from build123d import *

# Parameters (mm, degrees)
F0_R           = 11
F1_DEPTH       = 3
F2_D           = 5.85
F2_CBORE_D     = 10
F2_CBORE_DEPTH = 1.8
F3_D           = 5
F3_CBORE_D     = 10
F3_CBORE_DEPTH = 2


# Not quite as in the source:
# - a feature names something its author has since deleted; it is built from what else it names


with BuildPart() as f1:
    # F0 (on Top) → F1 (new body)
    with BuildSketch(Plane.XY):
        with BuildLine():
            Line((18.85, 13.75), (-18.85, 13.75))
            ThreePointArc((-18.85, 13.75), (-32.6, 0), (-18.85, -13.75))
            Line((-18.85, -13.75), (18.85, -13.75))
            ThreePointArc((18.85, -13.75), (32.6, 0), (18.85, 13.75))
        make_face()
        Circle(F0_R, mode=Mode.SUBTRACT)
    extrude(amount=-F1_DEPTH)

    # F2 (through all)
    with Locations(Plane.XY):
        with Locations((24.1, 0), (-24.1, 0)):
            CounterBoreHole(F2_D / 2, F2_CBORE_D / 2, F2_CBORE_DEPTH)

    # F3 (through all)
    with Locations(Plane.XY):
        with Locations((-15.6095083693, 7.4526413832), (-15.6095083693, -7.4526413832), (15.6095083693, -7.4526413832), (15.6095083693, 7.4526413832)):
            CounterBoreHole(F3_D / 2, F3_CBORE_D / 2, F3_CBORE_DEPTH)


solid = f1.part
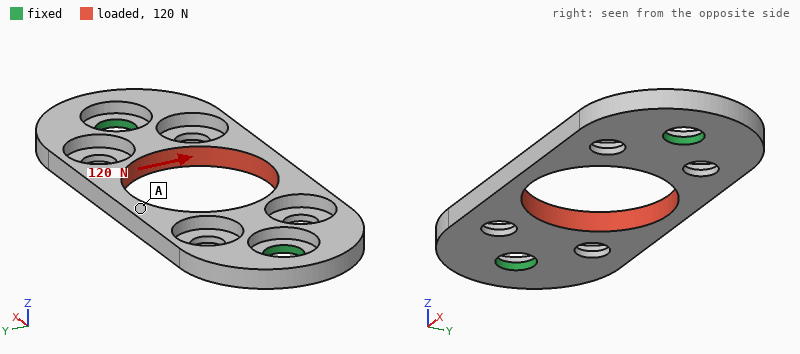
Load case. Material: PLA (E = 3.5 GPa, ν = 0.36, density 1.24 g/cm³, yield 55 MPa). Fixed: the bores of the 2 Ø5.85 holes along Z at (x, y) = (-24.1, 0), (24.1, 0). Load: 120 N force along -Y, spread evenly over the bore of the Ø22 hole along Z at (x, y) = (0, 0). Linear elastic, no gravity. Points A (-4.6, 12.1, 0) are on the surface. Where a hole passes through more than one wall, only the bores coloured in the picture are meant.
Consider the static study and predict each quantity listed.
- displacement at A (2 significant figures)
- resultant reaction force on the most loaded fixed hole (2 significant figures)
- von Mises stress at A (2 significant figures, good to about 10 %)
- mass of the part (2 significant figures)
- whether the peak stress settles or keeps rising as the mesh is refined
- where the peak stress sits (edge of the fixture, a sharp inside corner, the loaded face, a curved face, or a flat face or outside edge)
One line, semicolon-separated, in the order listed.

0.097 mm; 60 N; 1.7 MPa; 3.3 g; keeps rising; edge of the fixture
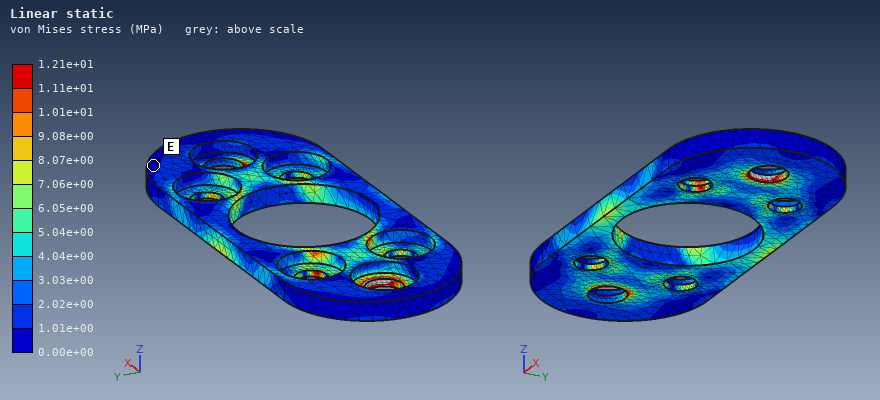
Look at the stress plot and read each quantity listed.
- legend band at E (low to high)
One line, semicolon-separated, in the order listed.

0.00e+00 to 1.01e+00 MPa
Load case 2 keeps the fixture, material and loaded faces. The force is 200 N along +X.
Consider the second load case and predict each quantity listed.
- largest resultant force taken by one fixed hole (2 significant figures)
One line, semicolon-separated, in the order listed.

100 N
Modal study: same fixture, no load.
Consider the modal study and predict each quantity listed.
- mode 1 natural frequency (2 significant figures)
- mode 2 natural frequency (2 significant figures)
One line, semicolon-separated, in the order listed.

1700 Hz; 1700 Hz
